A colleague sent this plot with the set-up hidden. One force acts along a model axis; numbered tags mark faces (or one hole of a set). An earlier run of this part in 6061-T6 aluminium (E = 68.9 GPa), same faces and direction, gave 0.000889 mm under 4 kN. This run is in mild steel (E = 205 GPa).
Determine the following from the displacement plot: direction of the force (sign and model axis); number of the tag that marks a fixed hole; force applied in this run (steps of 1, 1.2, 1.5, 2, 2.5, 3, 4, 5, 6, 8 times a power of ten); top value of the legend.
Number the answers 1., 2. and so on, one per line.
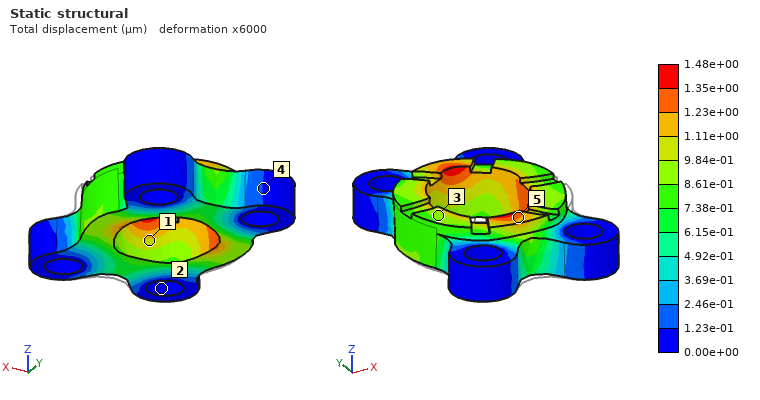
1. +Y
2. 2
3. 20 kN
4. 1.48e+00 µm
